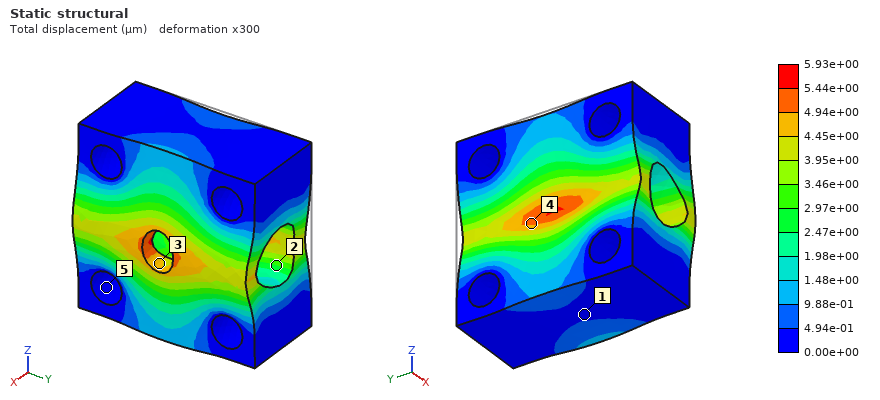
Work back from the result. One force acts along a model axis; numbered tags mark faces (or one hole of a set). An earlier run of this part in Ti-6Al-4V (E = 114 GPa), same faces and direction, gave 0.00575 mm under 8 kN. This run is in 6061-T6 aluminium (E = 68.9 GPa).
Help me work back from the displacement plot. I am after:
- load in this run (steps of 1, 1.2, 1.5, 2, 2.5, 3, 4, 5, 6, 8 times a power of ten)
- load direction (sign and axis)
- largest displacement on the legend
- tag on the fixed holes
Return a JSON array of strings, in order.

["5 kN", "+X", "5.93e+00 µm", "5"]
